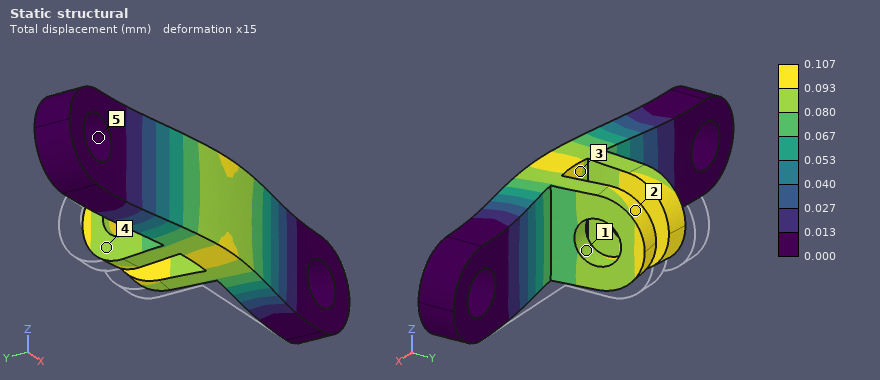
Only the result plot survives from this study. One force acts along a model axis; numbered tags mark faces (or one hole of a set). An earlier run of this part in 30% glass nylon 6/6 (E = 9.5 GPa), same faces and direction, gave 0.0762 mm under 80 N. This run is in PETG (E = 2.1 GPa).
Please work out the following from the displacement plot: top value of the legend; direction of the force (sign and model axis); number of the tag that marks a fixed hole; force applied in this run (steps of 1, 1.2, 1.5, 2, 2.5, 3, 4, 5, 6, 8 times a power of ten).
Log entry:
0.107 mm
-Y
5
25 N
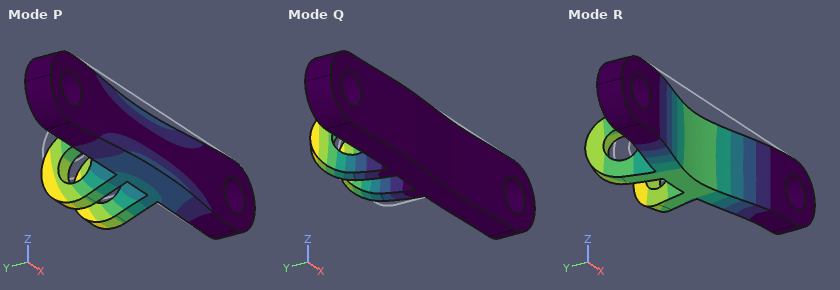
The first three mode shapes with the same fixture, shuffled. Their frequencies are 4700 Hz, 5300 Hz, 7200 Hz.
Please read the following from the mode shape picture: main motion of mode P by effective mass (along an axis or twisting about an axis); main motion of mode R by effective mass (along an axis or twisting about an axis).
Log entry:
along Z
along Y
